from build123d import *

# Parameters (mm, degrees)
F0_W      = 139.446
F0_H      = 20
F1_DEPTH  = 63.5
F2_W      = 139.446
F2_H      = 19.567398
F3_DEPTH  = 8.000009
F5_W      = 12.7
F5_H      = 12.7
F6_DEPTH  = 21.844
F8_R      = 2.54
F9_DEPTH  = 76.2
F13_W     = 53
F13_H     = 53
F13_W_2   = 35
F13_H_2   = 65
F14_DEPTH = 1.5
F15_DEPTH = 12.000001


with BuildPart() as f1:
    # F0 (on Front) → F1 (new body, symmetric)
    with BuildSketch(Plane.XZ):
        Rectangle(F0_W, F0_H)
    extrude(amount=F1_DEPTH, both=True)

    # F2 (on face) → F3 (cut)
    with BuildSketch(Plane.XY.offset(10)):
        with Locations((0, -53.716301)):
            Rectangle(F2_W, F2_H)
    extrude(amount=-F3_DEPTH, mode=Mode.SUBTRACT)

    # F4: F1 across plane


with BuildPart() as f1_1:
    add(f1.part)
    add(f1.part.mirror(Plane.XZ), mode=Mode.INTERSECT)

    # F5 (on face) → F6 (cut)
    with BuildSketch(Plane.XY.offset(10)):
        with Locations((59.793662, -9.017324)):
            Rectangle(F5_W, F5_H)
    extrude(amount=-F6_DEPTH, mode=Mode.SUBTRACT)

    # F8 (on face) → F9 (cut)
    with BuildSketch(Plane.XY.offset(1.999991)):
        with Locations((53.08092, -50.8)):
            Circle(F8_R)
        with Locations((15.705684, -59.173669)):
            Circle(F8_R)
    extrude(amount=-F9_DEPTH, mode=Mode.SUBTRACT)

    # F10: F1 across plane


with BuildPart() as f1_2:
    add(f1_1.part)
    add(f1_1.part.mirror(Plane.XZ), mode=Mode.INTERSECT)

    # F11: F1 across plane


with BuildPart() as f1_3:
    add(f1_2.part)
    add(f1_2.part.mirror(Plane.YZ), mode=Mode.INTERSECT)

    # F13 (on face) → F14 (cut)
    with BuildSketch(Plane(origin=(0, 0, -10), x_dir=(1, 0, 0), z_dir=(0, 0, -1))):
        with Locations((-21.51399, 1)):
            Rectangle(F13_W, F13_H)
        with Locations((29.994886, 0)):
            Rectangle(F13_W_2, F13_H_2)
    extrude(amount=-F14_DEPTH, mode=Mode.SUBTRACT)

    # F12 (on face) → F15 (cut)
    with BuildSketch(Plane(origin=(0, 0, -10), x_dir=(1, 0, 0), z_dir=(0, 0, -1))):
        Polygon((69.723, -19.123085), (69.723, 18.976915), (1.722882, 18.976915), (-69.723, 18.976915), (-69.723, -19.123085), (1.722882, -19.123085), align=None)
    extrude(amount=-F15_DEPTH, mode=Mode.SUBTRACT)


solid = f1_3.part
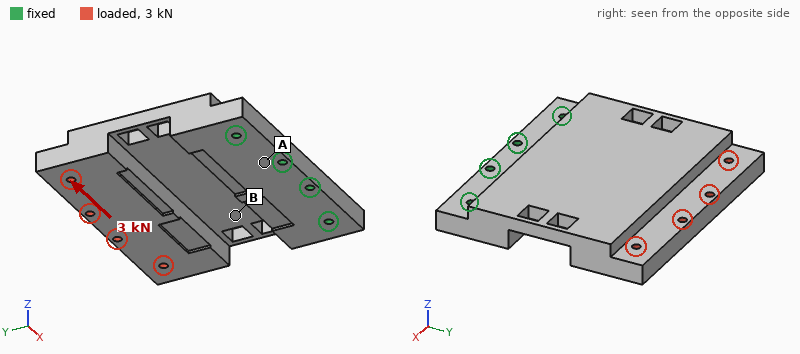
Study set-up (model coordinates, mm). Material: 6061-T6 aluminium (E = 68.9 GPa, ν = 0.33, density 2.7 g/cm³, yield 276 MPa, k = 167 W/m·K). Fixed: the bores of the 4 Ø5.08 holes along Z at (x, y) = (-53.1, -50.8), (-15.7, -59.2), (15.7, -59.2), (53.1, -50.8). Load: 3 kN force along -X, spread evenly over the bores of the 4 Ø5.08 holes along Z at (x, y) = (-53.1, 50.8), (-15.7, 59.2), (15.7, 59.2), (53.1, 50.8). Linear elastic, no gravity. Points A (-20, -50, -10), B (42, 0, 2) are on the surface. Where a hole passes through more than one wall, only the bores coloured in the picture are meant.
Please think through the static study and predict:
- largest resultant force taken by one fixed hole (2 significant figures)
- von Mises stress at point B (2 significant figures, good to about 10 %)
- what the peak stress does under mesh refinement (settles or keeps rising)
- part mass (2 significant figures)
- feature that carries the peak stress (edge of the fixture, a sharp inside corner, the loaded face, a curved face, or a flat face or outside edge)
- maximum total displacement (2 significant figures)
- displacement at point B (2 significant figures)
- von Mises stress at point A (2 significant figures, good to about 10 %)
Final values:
3.0 kN
16 MPa
keeps rising
640 g
edge of the fixture
93 µm
35 µm
6.7 MPa
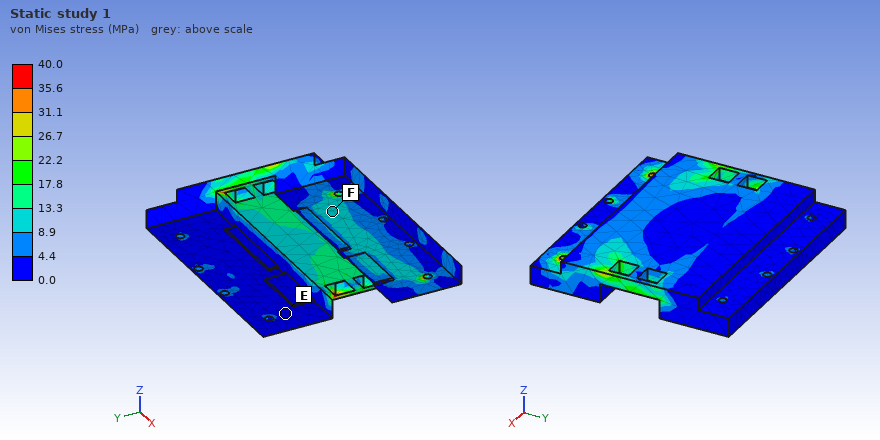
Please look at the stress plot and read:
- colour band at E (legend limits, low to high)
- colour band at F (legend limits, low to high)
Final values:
0.0 to 4.4 MPa
8.9 to 13.3 MPa
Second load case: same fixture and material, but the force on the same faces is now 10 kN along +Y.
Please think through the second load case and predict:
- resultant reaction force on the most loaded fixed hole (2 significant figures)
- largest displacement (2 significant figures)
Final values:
2.7 kN
0.81 mm
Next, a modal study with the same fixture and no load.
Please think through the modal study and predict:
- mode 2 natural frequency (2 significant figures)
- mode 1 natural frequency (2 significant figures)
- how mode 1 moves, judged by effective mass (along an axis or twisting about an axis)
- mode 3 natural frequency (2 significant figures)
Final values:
1300 Hz
510 Hz
along Z
2600 Hz
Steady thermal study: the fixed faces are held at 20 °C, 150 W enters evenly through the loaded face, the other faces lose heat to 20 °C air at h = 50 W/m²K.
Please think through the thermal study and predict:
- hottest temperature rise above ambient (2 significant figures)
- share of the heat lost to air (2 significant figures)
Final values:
59 K
40 %
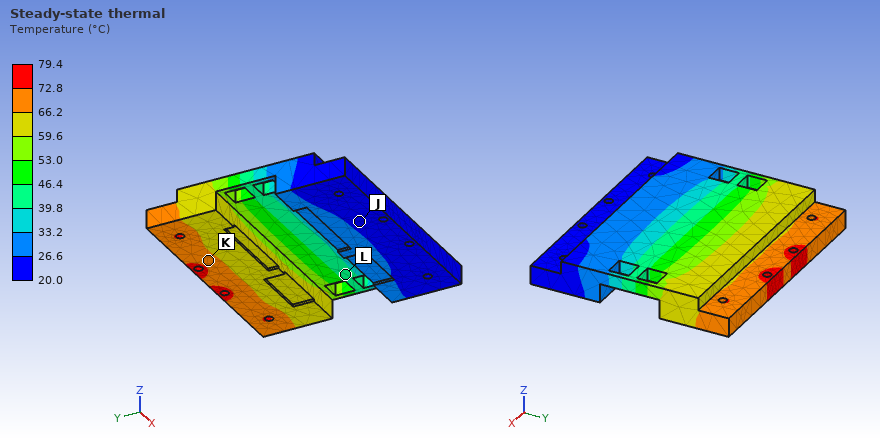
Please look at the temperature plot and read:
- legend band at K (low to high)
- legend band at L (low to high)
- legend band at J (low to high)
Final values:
66.2 to 72.8 °C
39.8 to 46.4 °C
20.0 to 26.6 °C
